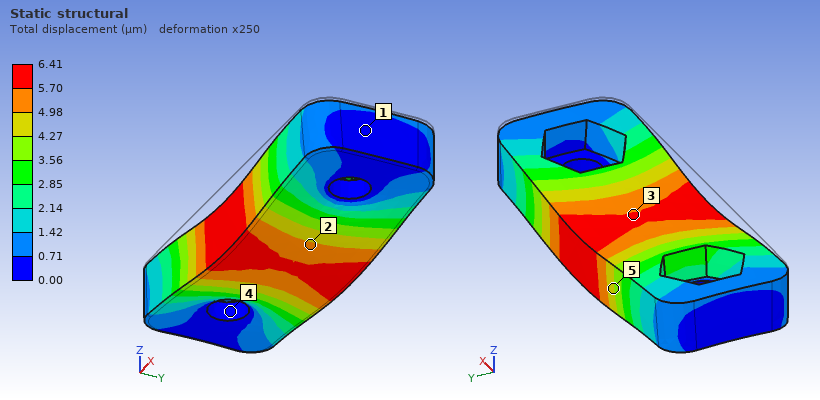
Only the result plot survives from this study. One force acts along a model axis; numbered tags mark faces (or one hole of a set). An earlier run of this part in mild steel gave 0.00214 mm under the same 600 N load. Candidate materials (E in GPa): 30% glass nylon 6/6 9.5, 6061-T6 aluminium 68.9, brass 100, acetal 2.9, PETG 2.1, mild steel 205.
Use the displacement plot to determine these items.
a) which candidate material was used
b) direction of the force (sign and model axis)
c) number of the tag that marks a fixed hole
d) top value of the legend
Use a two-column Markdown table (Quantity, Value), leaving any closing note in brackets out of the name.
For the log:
| Quantity | Value |
|---|---|
| which candidate material was used | 6061-T6 aluminium |
| direction of the force | -Z |
| number of the tag that marks a fixed hole | 4 |
| top value of the legend | 6.41 µm |
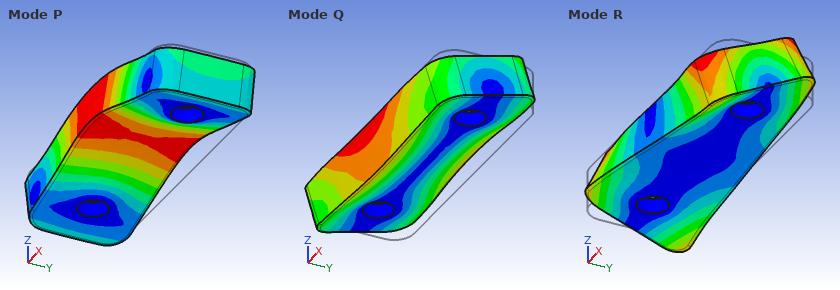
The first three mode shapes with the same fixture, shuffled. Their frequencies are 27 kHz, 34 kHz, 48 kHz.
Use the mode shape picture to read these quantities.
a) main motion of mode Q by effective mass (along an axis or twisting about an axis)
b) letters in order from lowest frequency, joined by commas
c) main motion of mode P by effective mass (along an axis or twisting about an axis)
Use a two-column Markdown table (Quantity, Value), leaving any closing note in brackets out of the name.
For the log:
| Quantity | Value |
|---|---|
| main motion of mode Q by effective mass | along Y |
| letters in order from lowest frequency, joined by commas | Q, P, R |
| main motion of mode P by effective mass | along Z |
